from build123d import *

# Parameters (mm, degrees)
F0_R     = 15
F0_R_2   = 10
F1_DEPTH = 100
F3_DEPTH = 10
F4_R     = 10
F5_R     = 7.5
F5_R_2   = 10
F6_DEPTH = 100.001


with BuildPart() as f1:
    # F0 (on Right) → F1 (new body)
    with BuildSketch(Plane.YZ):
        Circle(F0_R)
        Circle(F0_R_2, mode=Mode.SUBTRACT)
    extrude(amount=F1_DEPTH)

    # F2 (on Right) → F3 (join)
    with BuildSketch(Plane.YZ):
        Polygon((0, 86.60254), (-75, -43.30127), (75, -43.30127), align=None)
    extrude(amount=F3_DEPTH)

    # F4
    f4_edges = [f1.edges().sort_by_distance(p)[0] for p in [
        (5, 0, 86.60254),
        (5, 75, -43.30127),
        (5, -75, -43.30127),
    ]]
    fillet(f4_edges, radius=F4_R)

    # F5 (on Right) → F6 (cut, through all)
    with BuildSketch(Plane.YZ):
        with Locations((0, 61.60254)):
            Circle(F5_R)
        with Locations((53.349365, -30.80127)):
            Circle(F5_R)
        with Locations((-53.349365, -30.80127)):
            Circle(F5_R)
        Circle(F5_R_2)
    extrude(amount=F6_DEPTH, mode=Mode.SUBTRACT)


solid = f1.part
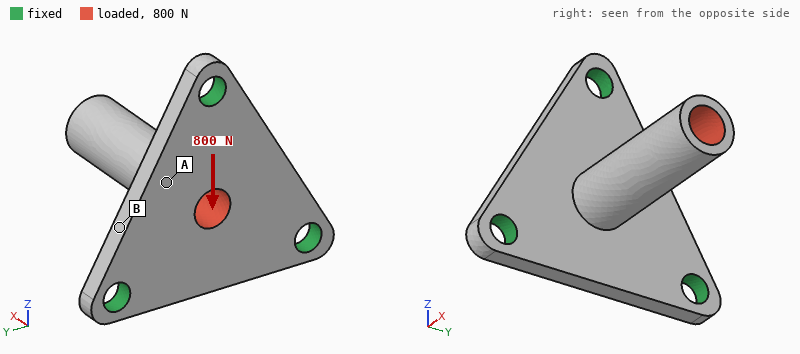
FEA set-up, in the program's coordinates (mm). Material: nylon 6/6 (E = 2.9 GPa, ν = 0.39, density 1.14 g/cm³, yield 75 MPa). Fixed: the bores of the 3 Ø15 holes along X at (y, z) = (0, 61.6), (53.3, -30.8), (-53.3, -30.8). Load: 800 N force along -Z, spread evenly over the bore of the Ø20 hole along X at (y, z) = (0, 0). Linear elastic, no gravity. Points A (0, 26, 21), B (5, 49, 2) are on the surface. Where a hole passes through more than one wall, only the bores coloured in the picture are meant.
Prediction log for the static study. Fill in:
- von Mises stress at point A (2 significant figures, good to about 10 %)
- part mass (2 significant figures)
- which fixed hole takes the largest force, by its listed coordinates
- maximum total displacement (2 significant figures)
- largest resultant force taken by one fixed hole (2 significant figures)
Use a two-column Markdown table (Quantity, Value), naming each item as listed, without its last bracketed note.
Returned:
| Quantity | Value |
|---|---|
| von Mises stress at point A | 6.1 MPa |
| part mass | 140 g |
| which fixed hole takes the largest force, by its listed coordinates | (0, 61.6) |
| maximum total displacement | 2.4 mm |
| largest resultant force taken by one fixed hole | 620 N |
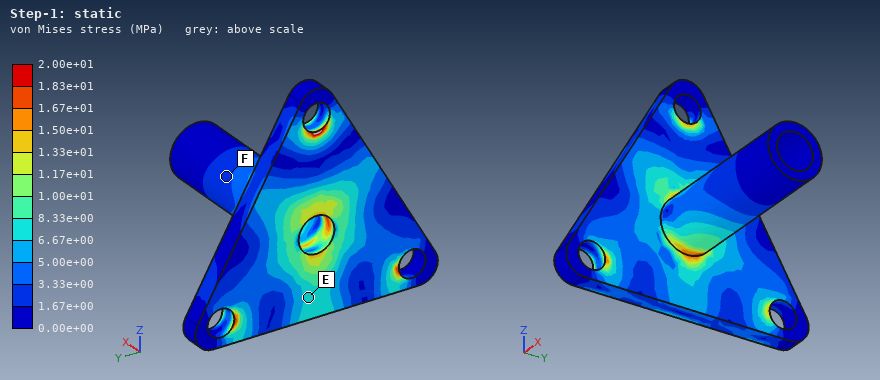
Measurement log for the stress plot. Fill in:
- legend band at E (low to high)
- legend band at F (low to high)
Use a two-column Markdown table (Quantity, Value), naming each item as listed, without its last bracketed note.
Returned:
| Quantity | Value |
|---|---|
| legend band at E | 6.67e+00 to 8.33e+00 MPa |
| legend band at F | 1.67e+00 to 3.33e+00 MPa |
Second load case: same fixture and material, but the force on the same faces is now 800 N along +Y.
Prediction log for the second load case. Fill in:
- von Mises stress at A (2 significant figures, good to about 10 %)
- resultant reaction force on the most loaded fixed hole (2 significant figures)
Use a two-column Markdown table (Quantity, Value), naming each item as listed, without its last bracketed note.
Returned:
| Quantity | Value |
|---|---|
| von Mises stress at A | 5.7 MPa |
| resultant reaction force on the most loaded fixed hole | 540 N |
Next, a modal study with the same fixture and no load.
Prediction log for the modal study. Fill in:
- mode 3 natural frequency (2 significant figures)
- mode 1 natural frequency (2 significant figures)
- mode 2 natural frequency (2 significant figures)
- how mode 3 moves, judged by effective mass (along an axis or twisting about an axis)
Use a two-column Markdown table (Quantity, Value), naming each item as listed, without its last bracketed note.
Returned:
| Quantity | Value |
|---|---|
| mode 3 natural frequency | 1000 Hz |
| mode 1 natural frequency | 530 Hz |
| mode 2 natural frequency | 530 Hz |
| how mode 3 moves, judged by effective mass | along X |
